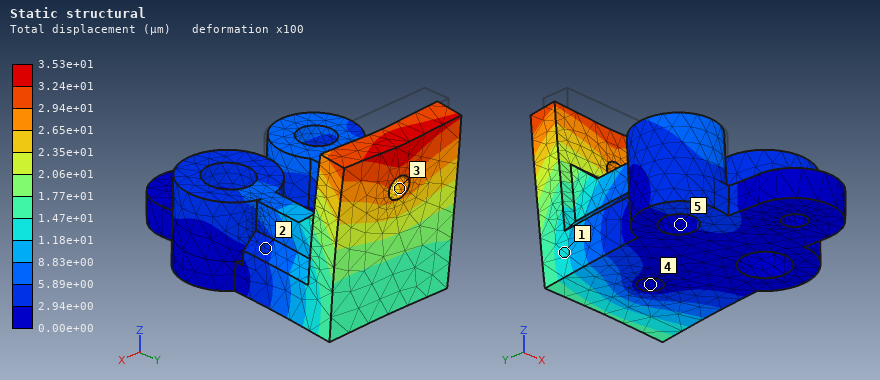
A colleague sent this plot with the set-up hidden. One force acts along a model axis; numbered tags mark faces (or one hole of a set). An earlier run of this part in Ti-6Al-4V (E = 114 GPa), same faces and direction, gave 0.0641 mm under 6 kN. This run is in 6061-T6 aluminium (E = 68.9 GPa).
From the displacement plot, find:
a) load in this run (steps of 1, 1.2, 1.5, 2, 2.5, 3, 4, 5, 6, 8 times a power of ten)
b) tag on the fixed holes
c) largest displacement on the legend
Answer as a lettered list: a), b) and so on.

a) 2 kN
b) 4
c) 3.53e+01 µm
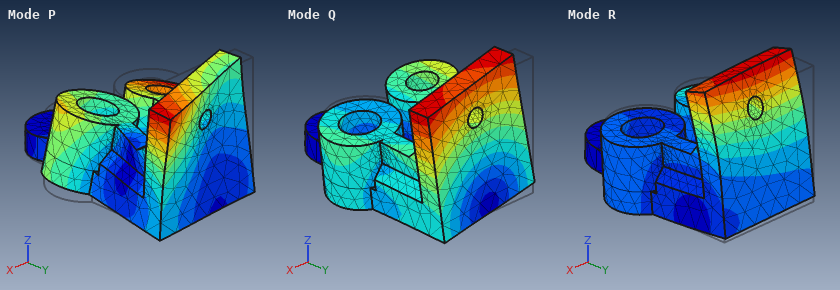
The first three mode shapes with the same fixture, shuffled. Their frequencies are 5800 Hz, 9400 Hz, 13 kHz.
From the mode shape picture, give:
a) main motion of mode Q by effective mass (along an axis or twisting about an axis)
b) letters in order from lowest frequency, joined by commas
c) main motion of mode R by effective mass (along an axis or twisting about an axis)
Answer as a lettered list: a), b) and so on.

a) along X
b) Q, R, P
c) along Y
